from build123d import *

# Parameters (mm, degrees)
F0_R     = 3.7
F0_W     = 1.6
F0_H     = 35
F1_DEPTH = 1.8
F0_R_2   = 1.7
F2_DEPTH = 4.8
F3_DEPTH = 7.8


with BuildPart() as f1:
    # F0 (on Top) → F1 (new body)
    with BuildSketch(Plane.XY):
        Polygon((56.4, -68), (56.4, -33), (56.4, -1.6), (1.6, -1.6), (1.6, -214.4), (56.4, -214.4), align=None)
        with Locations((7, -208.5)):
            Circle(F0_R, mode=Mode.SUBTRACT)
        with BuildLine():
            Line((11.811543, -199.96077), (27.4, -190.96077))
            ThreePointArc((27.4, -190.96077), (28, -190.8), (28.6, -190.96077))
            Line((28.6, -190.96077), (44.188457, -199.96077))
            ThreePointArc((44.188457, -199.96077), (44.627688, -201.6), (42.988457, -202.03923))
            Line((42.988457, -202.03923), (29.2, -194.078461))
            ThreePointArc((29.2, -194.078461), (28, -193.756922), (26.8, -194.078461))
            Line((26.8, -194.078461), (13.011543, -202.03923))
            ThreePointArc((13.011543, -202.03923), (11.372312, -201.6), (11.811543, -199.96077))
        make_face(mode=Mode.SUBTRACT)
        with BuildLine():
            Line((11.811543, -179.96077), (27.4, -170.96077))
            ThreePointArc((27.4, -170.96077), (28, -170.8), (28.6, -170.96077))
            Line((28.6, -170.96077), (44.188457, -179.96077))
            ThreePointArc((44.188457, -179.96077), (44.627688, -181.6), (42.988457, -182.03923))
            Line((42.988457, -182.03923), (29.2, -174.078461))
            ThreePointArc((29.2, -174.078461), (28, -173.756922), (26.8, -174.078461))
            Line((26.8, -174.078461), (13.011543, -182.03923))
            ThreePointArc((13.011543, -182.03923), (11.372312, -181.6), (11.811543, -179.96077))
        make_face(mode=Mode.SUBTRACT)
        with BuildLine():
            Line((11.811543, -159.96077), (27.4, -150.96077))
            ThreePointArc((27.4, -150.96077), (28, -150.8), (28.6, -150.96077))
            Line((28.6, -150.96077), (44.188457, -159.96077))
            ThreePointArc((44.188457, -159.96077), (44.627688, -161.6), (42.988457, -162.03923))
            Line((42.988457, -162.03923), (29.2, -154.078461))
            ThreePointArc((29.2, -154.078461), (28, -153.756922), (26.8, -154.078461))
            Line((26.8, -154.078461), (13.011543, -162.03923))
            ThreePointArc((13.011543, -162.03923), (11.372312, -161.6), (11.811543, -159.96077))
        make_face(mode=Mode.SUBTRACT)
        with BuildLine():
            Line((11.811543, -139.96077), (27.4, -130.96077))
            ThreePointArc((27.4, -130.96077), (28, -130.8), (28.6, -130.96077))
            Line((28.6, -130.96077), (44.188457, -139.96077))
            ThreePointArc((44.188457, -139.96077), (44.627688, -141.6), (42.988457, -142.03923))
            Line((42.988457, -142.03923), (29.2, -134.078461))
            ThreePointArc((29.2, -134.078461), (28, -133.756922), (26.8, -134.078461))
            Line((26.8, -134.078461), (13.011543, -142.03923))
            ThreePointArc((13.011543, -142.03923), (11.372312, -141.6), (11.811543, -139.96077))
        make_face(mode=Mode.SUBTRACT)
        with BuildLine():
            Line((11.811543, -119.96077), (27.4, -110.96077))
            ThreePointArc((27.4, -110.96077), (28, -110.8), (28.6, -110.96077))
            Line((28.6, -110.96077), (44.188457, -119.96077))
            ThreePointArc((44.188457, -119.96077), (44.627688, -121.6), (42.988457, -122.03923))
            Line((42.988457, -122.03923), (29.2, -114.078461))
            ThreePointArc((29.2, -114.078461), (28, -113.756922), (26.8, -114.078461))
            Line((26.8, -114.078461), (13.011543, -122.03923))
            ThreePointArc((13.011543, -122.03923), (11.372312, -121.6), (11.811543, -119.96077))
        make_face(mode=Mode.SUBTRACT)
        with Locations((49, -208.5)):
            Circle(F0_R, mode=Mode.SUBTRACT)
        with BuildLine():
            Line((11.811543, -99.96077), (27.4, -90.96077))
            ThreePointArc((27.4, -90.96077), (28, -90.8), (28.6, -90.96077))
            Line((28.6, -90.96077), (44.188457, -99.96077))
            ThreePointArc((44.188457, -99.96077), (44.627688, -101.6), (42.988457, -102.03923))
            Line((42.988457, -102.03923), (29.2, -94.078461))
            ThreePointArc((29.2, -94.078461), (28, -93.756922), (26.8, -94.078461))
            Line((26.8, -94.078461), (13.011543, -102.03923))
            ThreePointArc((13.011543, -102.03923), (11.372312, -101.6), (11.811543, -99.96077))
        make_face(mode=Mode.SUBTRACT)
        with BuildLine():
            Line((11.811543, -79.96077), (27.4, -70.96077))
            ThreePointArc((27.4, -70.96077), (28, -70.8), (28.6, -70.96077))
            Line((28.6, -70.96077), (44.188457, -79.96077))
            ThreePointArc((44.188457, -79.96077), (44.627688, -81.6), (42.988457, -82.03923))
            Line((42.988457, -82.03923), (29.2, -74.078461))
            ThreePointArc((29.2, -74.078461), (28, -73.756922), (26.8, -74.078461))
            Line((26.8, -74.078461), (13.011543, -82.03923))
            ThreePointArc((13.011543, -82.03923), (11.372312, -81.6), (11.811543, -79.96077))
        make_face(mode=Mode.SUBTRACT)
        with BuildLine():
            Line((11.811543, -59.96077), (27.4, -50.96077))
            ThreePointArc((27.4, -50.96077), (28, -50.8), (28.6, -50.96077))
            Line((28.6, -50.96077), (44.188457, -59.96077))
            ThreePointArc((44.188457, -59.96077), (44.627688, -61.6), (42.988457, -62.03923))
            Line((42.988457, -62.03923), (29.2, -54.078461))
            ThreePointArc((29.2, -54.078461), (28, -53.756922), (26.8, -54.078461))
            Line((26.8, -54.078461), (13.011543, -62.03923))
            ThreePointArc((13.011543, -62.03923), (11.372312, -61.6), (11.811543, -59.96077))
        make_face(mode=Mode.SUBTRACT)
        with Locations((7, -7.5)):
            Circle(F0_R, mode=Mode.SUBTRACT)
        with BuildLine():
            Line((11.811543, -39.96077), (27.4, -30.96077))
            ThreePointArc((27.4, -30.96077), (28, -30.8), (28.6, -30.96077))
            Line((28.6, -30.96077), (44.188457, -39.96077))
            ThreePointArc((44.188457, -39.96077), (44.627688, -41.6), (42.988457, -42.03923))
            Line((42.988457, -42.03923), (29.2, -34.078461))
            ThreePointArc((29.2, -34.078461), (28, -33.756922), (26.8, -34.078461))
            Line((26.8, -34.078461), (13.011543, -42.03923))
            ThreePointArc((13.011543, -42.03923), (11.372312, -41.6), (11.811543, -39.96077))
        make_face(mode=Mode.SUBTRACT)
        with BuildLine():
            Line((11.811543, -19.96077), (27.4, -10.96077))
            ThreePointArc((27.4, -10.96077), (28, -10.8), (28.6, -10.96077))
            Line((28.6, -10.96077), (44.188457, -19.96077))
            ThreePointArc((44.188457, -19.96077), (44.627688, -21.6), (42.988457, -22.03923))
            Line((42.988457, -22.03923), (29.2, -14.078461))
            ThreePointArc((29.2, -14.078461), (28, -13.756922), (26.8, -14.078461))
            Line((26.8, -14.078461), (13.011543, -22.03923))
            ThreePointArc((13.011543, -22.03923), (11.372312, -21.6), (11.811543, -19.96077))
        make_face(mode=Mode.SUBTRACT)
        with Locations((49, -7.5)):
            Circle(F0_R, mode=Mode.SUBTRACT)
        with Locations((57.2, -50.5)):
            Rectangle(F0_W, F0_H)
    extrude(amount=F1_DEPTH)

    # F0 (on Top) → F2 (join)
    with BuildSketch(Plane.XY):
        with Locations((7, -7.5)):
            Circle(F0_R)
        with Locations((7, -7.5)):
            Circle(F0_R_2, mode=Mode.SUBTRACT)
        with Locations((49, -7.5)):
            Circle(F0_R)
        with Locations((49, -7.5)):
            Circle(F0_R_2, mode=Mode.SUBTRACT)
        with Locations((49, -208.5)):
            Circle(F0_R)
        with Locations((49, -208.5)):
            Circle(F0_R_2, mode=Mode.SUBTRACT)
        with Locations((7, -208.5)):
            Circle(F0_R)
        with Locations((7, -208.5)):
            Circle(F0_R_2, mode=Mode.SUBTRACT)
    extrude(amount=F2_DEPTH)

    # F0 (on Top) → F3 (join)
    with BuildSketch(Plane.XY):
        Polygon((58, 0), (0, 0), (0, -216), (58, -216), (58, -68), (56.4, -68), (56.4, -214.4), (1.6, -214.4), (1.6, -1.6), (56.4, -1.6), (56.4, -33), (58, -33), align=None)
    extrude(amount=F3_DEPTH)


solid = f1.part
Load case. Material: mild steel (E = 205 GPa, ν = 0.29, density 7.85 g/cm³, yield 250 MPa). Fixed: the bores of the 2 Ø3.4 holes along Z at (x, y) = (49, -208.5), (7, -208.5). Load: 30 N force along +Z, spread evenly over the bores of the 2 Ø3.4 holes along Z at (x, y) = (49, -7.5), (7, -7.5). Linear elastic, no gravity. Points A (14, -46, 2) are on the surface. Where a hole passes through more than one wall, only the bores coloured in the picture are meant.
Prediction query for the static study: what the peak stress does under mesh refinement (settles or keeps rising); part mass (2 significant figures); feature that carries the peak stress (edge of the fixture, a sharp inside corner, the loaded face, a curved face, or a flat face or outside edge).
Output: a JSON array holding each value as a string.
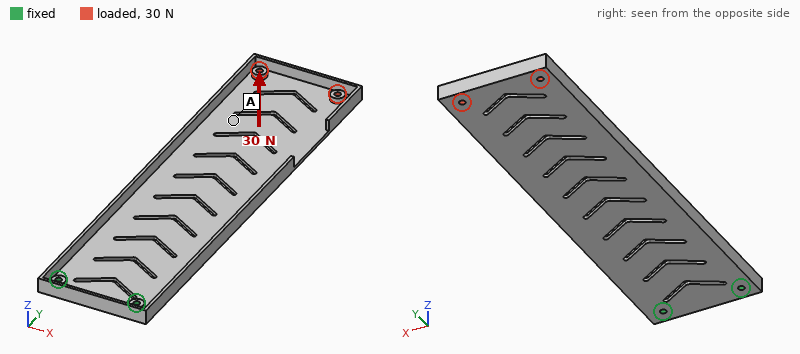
["keeps rising", "210 g", "a sharp inside corner"]
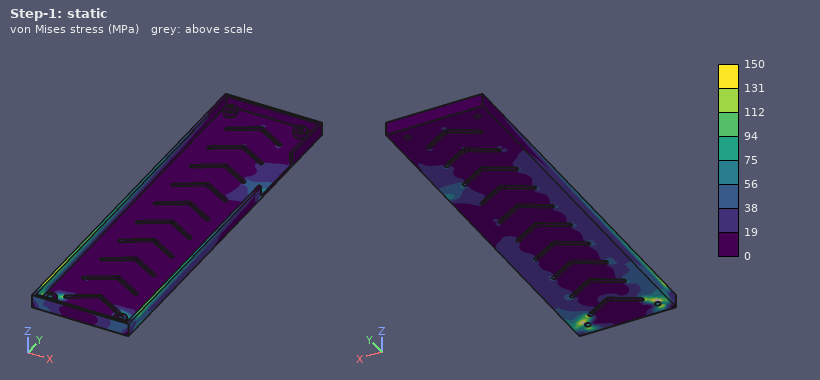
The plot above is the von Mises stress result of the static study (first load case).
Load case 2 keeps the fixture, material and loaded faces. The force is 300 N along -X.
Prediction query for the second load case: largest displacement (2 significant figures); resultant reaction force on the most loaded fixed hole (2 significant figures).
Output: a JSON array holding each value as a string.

["0.57 mm", "1.3 kN"]
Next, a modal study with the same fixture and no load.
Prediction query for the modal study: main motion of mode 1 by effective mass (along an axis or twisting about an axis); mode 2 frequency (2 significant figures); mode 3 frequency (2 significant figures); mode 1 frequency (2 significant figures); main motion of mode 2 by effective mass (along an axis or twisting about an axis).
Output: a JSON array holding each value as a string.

["along Z", "240 Hz", "420 Hz", "80 Hz", "twisting about Y"]
